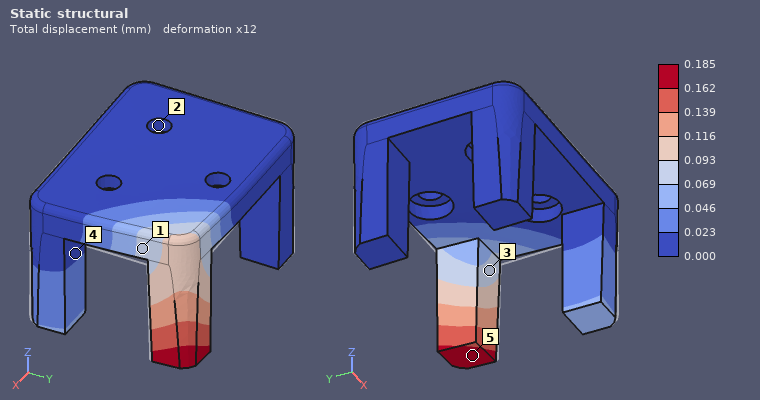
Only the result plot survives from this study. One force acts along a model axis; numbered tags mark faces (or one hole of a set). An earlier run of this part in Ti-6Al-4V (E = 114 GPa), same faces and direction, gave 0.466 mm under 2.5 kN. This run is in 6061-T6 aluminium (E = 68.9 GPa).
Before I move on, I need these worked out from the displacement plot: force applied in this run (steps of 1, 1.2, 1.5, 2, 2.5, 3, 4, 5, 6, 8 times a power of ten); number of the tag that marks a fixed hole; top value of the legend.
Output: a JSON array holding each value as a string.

["600 N", "2", "0.185 mm"]
